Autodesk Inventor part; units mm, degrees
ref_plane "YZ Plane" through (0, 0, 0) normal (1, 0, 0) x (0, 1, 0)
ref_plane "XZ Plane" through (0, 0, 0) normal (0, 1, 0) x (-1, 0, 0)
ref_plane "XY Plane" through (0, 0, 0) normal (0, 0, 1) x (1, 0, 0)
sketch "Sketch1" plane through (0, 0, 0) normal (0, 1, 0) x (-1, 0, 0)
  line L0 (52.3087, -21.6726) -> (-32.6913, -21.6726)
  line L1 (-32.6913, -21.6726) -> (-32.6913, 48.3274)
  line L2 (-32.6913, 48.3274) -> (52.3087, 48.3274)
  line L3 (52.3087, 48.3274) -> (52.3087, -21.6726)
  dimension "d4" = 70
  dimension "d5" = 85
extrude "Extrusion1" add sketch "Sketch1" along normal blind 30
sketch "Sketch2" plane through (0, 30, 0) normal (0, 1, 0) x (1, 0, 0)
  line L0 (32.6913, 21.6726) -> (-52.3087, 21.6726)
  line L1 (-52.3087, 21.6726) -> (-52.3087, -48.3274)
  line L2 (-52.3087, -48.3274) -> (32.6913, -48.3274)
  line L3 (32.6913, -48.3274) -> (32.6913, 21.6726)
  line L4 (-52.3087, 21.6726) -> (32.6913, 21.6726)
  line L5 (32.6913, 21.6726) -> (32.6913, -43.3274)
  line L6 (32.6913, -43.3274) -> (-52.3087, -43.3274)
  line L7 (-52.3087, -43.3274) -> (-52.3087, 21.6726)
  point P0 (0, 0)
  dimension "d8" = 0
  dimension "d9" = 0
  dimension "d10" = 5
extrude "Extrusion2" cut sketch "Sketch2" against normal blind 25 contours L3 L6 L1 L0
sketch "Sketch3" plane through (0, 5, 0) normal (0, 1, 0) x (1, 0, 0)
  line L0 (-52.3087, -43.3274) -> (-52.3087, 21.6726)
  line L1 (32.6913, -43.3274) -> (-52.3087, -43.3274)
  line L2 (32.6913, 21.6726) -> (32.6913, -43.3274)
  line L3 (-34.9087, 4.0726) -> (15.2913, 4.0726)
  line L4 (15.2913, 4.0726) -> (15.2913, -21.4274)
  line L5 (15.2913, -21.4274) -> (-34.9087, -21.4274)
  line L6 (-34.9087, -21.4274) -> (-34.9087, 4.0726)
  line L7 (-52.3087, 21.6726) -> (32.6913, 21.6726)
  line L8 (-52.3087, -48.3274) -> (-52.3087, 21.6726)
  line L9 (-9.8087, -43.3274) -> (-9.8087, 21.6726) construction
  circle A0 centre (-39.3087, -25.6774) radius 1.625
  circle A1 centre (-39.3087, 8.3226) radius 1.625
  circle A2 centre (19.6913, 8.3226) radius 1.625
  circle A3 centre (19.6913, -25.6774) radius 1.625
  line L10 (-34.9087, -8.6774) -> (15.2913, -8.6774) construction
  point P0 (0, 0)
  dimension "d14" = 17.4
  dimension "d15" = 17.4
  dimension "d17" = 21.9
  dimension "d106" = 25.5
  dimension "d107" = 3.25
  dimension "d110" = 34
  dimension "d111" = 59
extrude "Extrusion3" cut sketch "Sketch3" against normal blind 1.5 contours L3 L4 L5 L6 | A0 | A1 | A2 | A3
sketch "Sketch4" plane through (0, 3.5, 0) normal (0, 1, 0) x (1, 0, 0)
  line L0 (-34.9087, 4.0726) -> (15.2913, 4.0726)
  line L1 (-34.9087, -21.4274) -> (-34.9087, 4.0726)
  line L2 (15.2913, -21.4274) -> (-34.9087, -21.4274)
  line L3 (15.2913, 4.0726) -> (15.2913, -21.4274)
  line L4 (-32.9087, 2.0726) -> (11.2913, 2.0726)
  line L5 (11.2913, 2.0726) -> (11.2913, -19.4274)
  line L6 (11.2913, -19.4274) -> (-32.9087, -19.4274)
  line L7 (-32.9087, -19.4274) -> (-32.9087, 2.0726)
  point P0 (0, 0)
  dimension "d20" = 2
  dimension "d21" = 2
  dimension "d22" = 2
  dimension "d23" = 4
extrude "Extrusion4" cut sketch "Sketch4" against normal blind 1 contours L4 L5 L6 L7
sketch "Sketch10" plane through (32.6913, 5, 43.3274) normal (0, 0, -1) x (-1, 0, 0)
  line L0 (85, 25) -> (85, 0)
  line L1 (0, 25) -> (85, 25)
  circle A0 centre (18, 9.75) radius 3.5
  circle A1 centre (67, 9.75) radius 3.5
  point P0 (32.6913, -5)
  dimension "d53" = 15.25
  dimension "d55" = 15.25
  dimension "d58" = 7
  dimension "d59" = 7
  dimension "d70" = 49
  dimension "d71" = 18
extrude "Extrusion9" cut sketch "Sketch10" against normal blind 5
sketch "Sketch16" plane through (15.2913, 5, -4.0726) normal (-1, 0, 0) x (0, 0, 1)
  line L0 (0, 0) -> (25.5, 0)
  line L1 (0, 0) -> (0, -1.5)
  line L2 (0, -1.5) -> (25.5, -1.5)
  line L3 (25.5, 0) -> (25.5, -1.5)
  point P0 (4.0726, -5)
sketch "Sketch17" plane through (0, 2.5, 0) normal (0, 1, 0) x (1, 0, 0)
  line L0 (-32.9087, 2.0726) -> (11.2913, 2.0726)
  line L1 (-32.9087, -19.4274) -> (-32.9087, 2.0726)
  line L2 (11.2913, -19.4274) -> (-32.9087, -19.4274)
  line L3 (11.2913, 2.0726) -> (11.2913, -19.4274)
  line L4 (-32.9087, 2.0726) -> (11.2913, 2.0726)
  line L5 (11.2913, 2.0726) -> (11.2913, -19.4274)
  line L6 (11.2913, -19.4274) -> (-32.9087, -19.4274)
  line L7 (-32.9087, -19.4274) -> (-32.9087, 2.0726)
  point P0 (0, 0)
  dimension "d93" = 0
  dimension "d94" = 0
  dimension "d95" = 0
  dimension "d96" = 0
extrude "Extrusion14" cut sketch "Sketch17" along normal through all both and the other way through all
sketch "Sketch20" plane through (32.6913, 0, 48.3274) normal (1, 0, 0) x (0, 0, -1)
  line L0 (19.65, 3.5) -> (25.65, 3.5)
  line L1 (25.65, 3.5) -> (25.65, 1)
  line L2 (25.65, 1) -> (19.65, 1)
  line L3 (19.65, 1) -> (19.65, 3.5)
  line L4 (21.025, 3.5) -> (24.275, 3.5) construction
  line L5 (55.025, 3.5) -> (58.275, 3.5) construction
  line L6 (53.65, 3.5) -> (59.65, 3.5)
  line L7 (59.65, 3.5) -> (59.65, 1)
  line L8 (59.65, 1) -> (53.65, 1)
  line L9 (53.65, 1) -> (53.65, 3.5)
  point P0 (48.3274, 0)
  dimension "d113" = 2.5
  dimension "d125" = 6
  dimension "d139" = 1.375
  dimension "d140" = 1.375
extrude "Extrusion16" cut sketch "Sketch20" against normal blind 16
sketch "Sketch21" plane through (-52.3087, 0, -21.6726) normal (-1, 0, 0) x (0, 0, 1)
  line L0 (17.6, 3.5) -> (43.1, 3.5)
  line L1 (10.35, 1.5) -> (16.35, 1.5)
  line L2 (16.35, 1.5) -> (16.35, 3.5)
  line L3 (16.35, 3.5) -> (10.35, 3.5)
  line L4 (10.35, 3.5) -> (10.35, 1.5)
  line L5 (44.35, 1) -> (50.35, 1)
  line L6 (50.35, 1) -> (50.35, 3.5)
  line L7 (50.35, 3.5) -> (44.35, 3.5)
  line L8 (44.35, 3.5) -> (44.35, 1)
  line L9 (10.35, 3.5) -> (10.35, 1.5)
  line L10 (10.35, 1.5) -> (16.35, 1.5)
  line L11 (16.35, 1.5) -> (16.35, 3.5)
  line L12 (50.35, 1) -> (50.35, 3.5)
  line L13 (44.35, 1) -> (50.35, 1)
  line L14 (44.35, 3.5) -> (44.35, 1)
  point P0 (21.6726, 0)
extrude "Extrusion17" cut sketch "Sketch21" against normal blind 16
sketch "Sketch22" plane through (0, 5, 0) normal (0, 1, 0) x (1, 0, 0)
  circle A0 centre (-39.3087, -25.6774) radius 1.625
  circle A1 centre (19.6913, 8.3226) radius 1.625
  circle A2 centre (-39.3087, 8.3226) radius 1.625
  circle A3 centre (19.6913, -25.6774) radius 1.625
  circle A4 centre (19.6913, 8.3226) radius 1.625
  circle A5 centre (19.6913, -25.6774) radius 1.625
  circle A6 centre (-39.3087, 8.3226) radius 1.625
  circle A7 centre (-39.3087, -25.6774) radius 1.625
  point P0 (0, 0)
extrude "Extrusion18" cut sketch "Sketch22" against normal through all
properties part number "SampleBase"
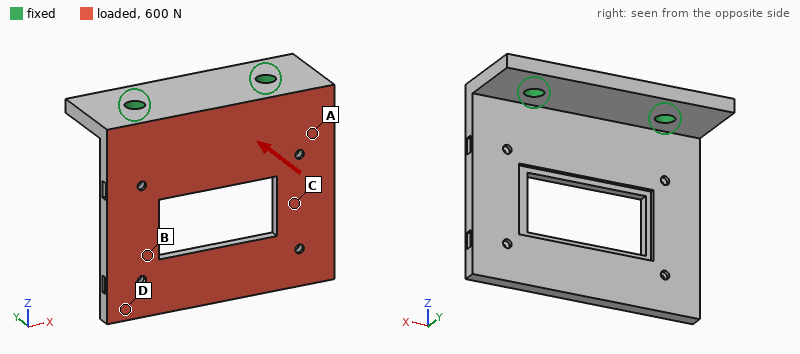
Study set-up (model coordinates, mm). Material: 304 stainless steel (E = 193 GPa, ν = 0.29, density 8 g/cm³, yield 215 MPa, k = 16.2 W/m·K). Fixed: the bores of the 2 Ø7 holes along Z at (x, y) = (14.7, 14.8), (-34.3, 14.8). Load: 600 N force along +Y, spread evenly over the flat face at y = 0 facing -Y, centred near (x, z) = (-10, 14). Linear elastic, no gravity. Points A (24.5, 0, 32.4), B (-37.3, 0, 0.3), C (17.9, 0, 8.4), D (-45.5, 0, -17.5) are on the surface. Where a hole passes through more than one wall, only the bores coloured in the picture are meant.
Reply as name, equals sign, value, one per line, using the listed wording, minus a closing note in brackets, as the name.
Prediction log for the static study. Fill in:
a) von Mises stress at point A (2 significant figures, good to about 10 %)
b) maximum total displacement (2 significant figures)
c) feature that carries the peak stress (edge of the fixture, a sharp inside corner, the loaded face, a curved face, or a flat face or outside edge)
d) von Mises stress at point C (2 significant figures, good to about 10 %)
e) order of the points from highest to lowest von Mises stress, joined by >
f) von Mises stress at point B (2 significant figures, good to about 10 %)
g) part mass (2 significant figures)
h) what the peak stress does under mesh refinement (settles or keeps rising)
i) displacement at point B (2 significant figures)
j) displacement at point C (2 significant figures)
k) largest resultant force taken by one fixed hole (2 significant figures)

von Mises stress at point A = 41 MPa
maximum total displacement = 0.27 mm
feature that carries the peak stress = edge of the fixture
von Mises stress at point C = 29 MPa
order of the points from highest to lowest von Mises stress, joined by > = A > C > B > D
von Mises stress at point B = 19 MPa
part mass = 270 g
what the peak stress does under mesh refinement = keeps rising
displacement at point B = 0.15 mm
displacement at point C = 0.12 mm
largest resultant force taken by one fixed hole = 300 N
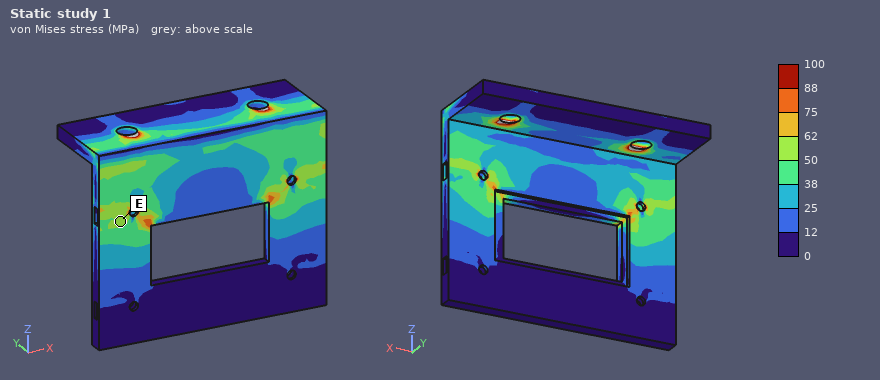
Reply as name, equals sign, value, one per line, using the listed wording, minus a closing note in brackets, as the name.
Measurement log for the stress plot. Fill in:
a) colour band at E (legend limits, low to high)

colour band at E = 50 to 62 MPa
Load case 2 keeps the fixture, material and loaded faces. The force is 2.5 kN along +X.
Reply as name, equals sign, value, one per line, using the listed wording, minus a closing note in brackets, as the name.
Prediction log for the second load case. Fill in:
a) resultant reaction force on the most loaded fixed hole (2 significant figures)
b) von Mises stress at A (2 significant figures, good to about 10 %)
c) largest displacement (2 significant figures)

resultant reaction force on the most loaded fixed hole = 2.0 kN
von Mises stress at A = 12 MPa
largest displacement = 47 µm
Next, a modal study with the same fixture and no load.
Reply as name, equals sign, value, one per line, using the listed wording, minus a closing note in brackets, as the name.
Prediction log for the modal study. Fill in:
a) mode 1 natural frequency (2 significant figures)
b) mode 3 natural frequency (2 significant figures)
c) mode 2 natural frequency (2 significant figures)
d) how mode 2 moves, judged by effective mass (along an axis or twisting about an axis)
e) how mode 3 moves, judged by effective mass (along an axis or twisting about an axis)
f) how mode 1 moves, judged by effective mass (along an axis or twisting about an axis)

mode 1 natural frequency = 660 Hz
mode 3 natural frequency = 3100 Hz
mode 2 natural frequency = 1400 Hz
how mode 2 moves, judged by effective mass = twisting about Z
how mode 3 moves, judged by effective mass = along X
how mode 1 moves, judged by effective mass = along Y
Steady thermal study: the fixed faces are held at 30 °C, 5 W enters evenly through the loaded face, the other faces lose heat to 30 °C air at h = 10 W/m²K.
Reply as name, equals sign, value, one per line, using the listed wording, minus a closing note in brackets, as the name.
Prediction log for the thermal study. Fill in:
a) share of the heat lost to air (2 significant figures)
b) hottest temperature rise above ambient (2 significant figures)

share of the heat lost to air = 36 %
hottest temperature rise above ambient = 31 K
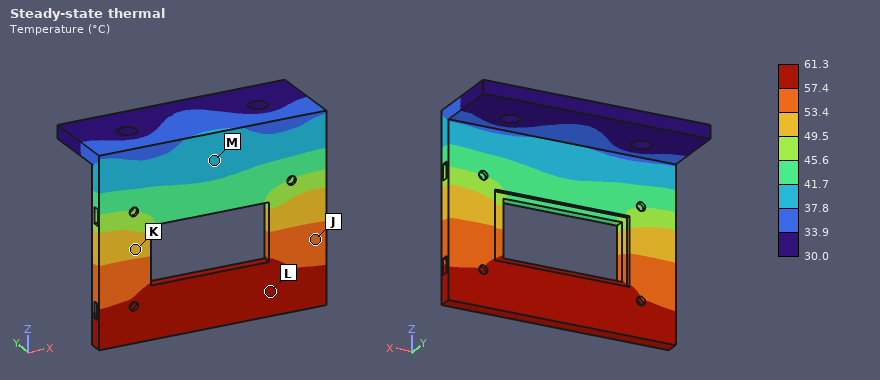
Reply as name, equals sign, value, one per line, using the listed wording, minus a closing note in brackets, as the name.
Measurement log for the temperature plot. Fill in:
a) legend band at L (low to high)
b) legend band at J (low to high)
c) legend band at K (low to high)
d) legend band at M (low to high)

legend band at L = 57.4 to 61.3 °C
legend band at J = 53.4 to 57.4 °C
legend band at K = 49.5 to 53.4 °C
legend band at M = 37.8 to 41.7 °C
